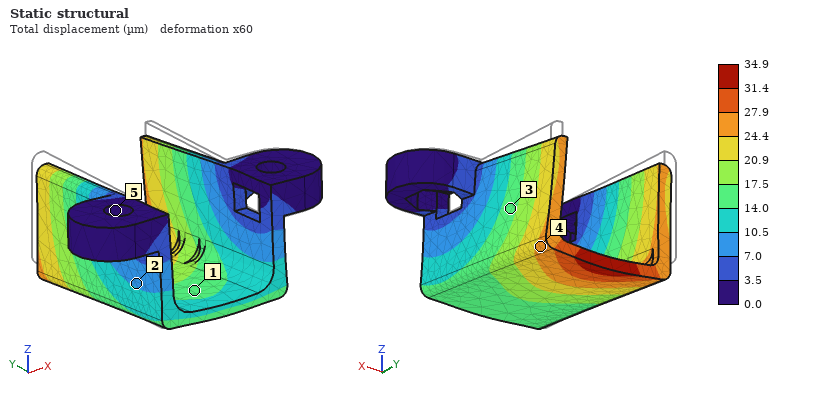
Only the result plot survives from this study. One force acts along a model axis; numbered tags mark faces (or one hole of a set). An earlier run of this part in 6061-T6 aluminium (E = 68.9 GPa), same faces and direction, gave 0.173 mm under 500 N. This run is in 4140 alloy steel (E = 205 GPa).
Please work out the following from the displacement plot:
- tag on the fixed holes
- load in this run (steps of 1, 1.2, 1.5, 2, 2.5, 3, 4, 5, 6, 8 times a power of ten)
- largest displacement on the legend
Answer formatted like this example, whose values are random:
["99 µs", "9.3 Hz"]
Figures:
["5", "300 N", "34.9 µm"]
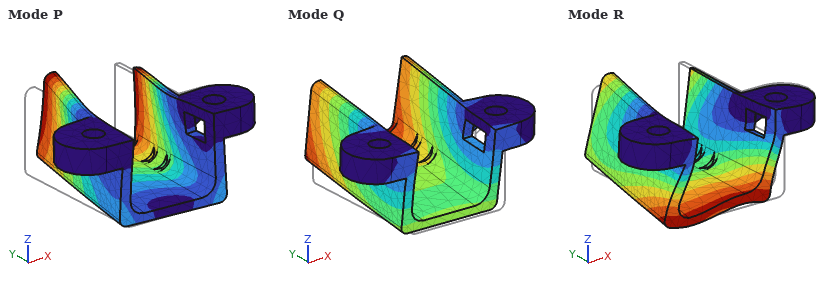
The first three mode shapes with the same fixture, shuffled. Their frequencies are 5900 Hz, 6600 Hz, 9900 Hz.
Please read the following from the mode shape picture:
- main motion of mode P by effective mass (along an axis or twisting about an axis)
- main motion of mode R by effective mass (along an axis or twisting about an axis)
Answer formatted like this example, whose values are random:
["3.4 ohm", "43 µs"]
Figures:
["along X", "along X"]
